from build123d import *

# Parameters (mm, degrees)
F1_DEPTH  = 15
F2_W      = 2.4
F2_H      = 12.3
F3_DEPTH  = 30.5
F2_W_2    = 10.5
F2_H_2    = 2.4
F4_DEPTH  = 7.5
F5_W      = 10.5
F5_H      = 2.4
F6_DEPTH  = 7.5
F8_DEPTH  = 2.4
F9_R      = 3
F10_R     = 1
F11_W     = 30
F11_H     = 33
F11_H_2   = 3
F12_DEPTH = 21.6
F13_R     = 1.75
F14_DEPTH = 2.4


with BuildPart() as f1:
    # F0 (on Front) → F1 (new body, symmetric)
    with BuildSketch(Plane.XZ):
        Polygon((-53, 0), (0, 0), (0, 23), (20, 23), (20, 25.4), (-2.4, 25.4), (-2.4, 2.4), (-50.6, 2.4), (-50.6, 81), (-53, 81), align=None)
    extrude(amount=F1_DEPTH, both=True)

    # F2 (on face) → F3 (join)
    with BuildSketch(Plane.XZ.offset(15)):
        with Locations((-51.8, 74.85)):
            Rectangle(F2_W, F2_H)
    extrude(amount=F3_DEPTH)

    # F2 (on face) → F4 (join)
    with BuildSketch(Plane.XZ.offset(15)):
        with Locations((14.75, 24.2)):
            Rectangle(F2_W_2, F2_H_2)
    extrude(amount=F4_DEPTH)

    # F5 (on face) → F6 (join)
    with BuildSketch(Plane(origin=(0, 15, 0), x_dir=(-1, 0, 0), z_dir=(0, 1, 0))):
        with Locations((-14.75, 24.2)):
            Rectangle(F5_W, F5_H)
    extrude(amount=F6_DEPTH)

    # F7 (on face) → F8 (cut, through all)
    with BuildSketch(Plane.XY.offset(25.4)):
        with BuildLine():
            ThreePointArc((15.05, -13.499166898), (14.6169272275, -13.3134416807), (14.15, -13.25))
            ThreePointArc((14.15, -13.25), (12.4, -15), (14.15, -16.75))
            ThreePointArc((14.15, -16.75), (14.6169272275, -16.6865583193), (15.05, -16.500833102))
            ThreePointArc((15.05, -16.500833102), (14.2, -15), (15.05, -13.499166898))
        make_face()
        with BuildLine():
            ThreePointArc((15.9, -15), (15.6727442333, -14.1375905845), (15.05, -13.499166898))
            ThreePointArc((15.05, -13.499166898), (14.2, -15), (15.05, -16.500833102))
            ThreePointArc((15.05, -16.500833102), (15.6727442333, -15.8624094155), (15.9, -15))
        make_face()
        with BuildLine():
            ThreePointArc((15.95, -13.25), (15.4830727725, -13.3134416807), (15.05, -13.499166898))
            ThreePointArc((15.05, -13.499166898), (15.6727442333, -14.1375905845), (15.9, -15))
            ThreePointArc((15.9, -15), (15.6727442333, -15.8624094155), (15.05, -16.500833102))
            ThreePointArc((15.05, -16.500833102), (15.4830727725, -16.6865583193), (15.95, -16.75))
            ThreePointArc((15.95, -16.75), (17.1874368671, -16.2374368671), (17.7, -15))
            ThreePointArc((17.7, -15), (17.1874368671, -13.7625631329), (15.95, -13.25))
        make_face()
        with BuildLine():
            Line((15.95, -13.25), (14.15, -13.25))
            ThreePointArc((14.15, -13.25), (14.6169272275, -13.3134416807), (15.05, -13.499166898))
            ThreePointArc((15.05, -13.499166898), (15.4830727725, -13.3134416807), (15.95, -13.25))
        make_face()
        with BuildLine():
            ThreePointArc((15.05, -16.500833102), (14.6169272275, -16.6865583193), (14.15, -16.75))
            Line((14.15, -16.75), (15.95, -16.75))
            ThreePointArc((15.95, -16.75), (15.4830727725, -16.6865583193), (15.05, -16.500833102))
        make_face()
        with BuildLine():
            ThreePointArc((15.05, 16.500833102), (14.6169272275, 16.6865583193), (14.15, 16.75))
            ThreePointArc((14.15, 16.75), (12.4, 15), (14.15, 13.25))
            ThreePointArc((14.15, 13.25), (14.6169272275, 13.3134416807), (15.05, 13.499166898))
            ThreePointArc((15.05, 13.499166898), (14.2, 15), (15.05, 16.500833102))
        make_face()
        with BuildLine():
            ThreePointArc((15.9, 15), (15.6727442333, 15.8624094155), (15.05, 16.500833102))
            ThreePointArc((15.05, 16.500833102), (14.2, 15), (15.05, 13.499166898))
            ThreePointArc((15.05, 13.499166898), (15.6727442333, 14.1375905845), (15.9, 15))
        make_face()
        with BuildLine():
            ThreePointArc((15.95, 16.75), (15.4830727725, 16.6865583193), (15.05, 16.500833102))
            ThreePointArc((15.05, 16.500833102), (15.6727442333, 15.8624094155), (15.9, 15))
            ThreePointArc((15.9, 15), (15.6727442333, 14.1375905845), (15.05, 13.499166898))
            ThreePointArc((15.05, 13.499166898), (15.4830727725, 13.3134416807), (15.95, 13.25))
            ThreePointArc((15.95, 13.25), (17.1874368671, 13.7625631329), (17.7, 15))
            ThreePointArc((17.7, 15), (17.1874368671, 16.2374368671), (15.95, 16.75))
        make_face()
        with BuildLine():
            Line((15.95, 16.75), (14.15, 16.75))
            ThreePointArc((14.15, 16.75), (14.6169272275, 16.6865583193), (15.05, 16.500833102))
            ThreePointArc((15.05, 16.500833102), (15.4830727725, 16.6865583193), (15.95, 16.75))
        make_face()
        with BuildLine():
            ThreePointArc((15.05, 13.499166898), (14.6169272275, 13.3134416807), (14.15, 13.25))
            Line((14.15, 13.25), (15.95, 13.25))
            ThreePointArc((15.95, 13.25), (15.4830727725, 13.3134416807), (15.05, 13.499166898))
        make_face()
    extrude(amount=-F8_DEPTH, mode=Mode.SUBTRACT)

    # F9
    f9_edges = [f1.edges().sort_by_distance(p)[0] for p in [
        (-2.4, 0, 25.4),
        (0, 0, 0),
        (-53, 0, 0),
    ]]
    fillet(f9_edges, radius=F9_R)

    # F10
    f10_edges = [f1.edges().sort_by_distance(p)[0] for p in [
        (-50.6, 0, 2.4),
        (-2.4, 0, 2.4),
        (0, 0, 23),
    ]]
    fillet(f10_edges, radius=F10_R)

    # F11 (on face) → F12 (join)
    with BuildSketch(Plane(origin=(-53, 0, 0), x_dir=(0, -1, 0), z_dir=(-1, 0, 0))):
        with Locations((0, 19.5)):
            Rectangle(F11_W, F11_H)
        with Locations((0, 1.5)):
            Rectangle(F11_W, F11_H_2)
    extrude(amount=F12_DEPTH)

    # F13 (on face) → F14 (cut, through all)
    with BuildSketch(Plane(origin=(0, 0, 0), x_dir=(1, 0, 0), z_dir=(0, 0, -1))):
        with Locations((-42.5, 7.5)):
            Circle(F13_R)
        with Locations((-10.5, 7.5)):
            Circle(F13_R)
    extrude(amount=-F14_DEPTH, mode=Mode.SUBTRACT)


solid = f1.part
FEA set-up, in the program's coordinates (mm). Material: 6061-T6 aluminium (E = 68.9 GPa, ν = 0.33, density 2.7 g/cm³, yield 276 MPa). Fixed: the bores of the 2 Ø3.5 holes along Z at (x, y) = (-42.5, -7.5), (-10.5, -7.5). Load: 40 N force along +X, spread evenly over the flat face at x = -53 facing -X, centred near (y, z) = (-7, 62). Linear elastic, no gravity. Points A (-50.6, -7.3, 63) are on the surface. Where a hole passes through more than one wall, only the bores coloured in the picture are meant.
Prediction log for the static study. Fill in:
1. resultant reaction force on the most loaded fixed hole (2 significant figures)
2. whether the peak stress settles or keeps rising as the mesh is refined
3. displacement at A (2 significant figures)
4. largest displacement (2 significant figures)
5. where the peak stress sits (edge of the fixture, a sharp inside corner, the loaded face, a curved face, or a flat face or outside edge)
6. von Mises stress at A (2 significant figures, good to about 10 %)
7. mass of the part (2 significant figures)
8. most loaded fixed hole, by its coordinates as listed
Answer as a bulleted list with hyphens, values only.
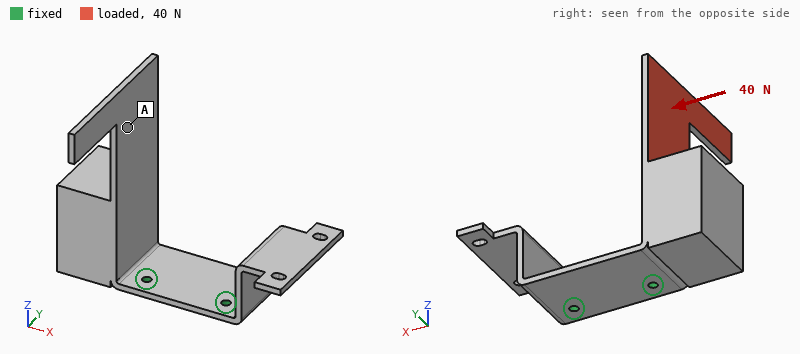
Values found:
- 43 N
- keeps rising
- 0.88 mm
- 1.4 mm
- edge of the fixture
- 11 MPa
- 100 g
- (-42.5, -7.5)
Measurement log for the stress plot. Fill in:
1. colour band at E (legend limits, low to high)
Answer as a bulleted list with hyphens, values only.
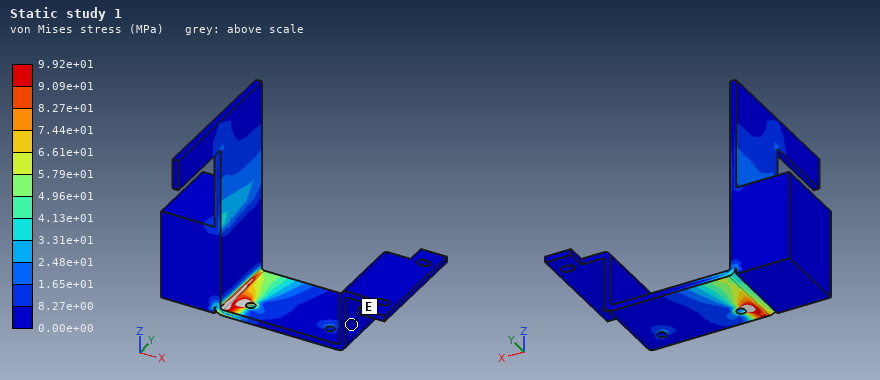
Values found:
- 0.00e+00 to 8.27e+00 MPa
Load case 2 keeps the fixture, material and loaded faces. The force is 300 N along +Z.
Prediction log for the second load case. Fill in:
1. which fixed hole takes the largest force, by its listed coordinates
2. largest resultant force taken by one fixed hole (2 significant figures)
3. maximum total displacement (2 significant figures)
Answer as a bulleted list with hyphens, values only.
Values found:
- (-42.5, -7.5)
- 320 N
- 0.77 mm
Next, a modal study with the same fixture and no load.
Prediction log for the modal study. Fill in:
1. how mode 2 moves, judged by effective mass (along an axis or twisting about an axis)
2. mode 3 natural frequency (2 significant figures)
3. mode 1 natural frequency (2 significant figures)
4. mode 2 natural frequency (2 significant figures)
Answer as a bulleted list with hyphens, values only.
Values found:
- along Y
- 790 Hz
- 230 Hz
- 380 Hz
